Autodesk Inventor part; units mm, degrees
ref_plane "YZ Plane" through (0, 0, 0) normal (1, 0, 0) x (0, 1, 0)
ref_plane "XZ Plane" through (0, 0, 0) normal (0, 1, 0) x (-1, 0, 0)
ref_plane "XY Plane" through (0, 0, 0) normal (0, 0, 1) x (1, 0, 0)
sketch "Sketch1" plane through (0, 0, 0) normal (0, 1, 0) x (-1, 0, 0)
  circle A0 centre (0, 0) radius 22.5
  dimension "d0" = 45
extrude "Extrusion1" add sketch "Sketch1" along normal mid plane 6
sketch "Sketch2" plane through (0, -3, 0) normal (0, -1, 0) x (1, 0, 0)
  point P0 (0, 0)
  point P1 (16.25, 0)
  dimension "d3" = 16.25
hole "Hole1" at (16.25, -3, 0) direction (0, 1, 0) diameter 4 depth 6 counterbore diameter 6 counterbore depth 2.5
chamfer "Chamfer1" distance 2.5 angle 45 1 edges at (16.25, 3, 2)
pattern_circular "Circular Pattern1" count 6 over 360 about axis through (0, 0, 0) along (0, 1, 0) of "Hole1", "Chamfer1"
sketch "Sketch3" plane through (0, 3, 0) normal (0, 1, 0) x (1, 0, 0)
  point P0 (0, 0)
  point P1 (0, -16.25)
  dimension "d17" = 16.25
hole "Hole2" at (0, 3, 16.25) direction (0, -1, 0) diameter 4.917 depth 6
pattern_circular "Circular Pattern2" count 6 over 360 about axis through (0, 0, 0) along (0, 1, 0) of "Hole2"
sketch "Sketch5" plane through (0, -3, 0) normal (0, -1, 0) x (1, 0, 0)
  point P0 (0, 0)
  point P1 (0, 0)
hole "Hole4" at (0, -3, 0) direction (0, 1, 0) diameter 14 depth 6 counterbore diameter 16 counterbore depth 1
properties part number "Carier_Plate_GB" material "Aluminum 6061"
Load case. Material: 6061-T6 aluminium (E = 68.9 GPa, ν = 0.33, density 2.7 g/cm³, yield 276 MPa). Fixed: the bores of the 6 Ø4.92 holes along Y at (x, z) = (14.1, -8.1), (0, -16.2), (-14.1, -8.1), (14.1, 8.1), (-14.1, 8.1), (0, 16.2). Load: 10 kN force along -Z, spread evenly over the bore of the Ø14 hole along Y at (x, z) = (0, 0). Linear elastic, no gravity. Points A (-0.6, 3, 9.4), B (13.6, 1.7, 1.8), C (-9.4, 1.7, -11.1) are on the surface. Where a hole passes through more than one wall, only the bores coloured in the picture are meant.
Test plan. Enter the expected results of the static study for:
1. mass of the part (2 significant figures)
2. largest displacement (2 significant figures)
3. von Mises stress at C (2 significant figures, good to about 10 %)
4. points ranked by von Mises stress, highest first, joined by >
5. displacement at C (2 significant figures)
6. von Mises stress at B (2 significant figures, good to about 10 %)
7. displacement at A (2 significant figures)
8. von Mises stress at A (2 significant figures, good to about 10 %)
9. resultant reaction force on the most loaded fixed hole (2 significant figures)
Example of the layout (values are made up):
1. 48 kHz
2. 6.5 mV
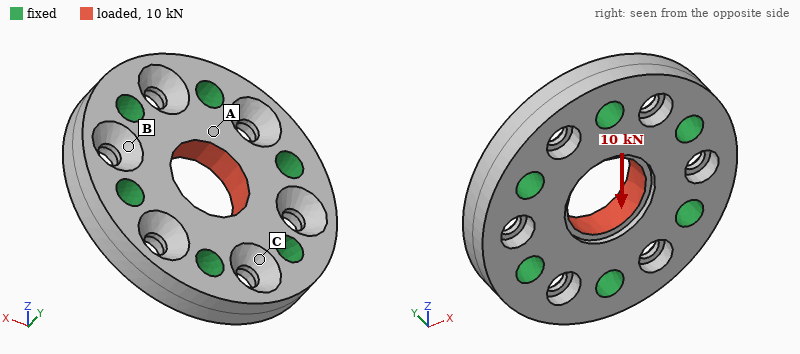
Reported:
1. 19 g
2. 6.9 µm
3. 33 MPa
4. A > C > B
5. 2.2 µm
6. 16 MPa
7. 4.4 µm
8. 60 MPa
9. 2.6 kN
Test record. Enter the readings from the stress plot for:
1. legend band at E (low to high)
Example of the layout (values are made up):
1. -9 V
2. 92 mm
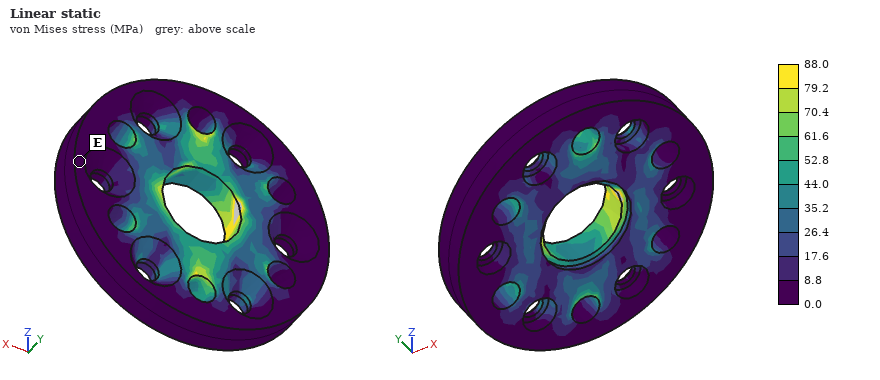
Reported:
1. 0.0 to 8.8 MPa
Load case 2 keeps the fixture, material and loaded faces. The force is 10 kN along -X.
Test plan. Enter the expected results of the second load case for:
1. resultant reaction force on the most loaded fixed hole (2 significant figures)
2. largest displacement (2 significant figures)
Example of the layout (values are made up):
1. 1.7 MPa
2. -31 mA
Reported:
1. 2.3 kN
2. 7.3 µm
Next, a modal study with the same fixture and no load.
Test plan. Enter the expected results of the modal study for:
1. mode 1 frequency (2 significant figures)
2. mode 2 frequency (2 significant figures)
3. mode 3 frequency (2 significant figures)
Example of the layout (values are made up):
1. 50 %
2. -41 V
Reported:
1. 62 kHz
2. 62 kHz
3. 63 kHz
